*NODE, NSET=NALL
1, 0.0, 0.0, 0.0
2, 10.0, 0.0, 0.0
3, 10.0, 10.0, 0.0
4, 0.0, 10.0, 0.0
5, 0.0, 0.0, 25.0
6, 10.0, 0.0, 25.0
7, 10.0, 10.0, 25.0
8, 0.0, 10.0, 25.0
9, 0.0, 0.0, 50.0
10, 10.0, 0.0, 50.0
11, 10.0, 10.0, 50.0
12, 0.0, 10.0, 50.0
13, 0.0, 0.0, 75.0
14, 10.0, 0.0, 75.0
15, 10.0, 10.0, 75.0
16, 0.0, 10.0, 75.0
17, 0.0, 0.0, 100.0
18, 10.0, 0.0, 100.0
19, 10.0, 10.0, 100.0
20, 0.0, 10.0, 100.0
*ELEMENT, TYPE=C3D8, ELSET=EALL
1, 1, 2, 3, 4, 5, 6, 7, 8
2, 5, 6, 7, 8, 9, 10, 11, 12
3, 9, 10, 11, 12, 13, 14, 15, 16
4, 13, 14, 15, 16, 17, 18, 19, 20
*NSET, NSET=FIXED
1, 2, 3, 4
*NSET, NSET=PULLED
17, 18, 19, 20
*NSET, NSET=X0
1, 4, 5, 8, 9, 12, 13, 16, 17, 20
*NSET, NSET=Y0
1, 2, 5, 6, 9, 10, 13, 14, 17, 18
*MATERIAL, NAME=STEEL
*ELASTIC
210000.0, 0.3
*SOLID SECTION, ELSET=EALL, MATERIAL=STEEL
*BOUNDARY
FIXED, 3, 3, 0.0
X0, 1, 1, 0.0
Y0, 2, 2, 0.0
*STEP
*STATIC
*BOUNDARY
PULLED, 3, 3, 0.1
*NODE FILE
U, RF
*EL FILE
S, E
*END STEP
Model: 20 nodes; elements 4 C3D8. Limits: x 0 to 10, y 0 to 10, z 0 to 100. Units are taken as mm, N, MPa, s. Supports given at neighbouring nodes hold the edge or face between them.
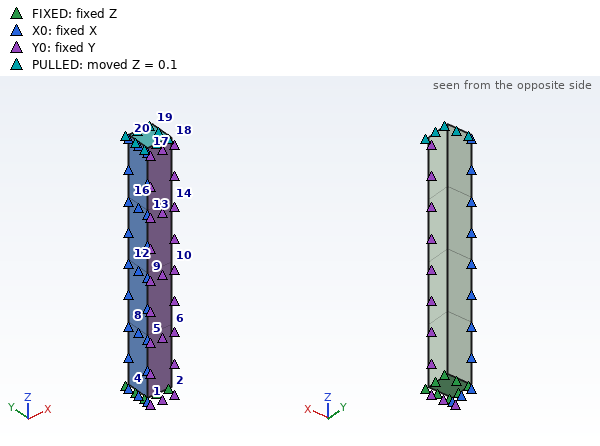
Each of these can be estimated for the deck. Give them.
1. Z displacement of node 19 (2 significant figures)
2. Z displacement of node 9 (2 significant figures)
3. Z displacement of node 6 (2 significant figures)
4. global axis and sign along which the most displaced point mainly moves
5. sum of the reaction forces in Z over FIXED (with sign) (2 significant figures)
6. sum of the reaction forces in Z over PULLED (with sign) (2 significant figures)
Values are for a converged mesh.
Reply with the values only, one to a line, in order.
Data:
0.10 mm
0.050 mm
0.025 mm
+Z
-21000 N
21000 N
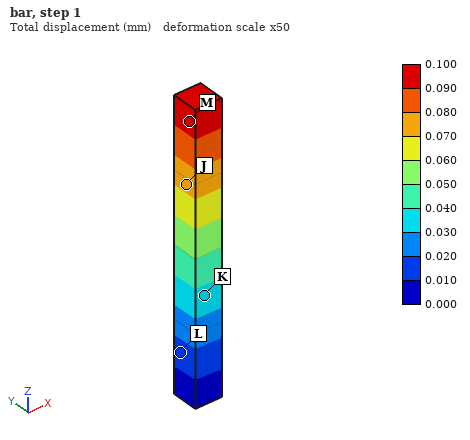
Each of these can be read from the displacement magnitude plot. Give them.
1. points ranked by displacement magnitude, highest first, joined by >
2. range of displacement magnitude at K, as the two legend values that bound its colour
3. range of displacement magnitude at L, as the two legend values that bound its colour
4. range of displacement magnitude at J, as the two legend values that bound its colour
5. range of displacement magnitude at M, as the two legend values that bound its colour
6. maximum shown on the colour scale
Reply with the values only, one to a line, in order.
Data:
M > J > K > L
0.030 to 0.040 mm
0.010 to 0.020 mm
0.070 to 0.080 mm
0.090 to 0.100 mm
0.100 mm
